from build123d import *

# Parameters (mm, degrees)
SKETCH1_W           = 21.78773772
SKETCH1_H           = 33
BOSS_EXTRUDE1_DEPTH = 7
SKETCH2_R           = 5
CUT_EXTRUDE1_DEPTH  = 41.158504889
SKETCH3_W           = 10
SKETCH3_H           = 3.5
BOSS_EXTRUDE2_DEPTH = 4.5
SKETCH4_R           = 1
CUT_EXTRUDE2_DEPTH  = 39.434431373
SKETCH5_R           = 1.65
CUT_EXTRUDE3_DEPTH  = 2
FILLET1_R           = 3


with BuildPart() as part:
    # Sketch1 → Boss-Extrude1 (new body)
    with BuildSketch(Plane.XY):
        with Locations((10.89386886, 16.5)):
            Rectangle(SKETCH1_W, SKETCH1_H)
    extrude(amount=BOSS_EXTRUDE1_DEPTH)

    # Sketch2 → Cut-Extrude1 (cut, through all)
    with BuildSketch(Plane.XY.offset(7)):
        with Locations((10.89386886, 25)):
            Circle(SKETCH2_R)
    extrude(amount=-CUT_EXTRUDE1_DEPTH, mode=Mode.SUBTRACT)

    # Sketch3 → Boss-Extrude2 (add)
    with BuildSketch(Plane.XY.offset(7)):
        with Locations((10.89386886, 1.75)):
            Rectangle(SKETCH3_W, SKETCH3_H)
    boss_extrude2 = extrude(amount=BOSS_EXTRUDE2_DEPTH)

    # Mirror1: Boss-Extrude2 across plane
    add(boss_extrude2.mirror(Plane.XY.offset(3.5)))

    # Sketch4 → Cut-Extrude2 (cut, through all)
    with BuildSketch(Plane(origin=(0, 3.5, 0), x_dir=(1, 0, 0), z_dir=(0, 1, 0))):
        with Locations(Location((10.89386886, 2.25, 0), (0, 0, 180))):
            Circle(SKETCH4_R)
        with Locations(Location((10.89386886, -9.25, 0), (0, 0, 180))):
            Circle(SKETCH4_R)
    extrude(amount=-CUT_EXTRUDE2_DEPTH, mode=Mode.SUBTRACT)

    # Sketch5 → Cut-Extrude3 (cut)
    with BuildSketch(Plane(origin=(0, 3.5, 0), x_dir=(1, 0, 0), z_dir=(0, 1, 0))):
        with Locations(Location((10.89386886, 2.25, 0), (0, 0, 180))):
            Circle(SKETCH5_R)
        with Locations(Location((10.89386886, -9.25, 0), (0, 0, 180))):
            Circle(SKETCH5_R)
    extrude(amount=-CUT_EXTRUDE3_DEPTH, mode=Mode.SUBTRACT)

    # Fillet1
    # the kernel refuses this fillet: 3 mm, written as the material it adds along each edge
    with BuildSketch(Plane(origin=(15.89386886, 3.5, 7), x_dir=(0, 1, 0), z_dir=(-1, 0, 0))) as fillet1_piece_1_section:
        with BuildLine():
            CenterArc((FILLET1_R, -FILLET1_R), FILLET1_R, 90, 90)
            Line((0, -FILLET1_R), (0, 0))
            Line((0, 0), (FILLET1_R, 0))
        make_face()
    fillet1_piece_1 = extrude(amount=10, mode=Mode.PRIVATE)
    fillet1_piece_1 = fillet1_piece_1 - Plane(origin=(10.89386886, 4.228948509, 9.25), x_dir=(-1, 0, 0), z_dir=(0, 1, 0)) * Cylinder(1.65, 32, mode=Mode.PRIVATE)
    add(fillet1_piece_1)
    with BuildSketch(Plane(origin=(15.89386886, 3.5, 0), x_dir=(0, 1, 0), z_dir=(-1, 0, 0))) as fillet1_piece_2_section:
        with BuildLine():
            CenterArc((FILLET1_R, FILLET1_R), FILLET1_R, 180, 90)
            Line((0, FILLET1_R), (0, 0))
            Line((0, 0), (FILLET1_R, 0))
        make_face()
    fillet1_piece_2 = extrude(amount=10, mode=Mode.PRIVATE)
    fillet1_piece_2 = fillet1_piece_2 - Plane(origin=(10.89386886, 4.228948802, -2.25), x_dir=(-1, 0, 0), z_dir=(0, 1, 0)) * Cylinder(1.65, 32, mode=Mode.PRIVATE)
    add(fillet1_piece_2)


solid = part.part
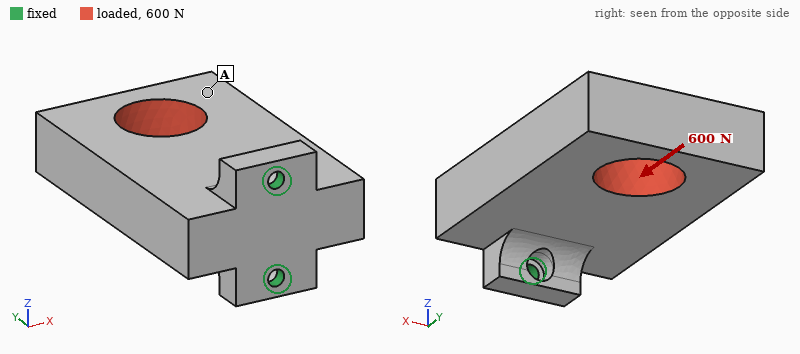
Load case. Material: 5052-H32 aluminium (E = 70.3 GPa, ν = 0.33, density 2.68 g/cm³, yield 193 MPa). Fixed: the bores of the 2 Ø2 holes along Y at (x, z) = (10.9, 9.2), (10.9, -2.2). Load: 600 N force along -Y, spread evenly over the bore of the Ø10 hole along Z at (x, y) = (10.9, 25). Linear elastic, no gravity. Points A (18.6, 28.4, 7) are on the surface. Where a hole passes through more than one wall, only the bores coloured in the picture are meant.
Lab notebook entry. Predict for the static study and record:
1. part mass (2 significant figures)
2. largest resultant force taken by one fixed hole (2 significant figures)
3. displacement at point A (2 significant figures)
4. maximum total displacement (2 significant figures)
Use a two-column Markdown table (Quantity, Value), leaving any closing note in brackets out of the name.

| Quantity | Value |
|---|---|
| part mass | 13 g |
| largest resultant force taken by one fixed hole | 330 N |
| displacement at point A | 4.6 µm |
| maximum total displacement | 6.3 µm |
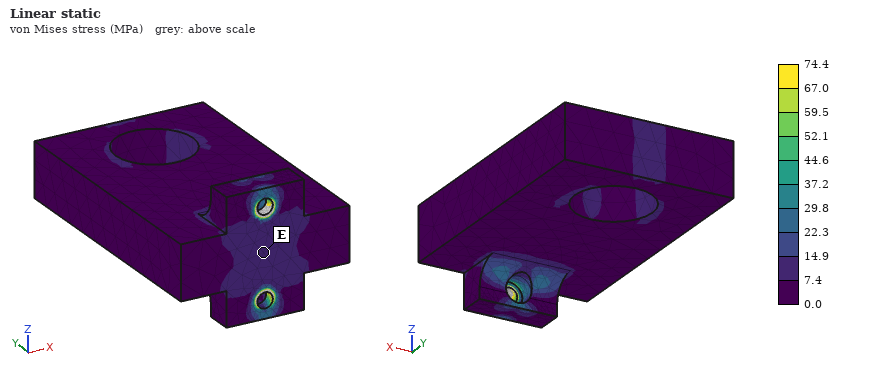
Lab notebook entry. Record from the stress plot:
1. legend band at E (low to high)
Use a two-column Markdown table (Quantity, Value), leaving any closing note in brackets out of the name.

| Quantity | Value |
|---|---|
| legend band at E | 7.4 to 14.9 MPa |
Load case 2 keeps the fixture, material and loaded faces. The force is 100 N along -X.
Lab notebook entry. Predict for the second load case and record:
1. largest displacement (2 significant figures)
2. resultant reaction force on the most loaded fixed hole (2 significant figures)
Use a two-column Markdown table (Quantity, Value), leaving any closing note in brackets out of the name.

| Quantity | Value |
|---|---|
| largest displacement | 0.15 mm |
| resultant reaction force on the most loaded fixed hole | 50 N |
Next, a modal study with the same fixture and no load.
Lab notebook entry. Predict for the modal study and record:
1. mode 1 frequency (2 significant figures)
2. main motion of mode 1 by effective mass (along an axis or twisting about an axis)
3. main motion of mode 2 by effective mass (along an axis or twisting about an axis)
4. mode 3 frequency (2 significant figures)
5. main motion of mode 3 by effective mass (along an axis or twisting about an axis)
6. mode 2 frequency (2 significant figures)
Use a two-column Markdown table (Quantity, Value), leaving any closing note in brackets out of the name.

| Quantity | Value |
|---|---|
| mode 1 frequency | 1800 Hz |
| main motion of mode 1 by effective mass | along X |
| main motion of mode 2 by effective mass | along Z |
| mode 3 frequency | 12 kHz |
| main motion of mode 3 by effective mass | twisting about Y |
| mode 2 frequency | 4800 Hz |
